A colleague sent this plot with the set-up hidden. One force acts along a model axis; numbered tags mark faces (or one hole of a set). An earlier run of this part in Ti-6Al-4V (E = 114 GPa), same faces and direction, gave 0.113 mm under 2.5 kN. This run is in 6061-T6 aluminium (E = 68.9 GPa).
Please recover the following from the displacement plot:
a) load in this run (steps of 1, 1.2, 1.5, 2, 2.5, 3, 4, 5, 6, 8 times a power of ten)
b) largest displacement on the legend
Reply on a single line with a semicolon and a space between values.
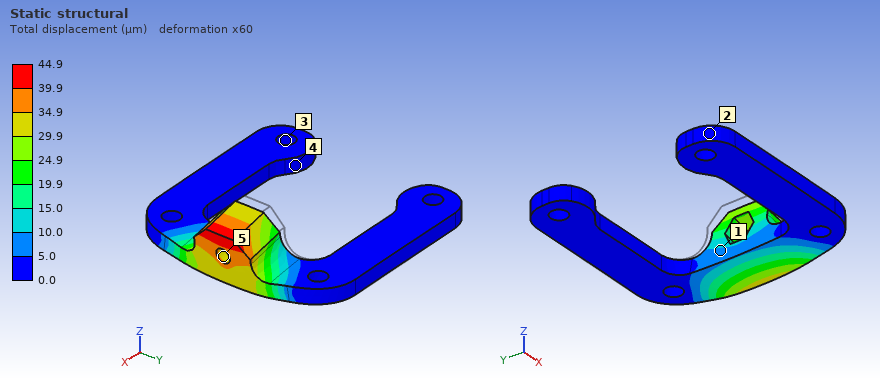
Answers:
600 N; 44.9 µm
